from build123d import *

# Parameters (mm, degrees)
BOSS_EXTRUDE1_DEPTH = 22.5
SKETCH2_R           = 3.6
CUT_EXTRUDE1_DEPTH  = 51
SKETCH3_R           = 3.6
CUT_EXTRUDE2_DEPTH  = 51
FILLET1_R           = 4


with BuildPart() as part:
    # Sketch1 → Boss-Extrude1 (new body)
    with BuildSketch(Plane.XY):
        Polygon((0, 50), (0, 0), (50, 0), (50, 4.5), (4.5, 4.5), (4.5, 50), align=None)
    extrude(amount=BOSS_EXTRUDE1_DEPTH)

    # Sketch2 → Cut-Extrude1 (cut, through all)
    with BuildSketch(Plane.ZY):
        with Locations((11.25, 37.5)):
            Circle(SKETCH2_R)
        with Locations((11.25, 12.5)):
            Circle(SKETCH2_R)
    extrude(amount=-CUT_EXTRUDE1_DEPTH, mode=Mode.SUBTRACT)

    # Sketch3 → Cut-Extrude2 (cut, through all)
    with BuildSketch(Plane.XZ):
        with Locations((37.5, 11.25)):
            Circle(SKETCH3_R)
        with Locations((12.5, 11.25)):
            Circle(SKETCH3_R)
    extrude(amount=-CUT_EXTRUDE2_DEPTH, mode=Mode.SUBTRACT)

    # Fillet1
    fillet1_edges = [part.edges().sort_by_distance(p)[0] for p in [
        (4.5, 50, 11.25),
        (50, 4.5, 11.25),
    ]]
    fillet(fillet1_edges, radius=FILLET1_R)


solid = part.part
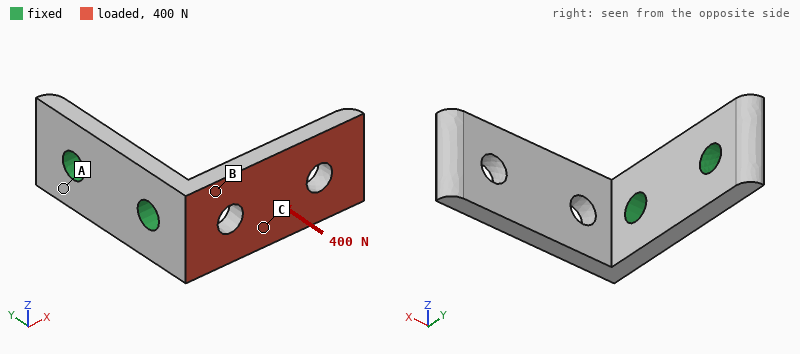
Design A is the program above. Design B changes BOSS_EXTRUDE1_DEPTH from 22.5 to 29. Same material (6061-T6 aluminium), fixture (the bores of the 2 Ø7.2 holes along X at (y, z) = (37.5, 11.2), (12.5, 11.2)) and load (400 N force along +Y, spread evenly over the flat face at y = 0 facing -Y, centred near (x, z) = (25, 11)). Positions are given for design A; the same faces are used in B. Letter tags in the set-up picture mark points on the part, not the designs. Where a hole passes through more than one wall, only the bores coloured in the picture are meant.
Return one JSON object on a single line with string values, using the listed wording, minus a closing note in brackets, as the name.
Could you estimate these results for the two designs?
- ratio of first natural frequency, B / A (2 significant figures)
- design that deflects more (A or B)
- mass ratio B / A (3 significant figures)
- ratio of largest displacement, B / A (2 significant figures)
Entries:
{"ratio of first natural frequency, B / A": "0.99", "design that deflects more": "A", "mass ratio B / A": "1.31", "ratio of largest displacement, B / A": "0.78"}
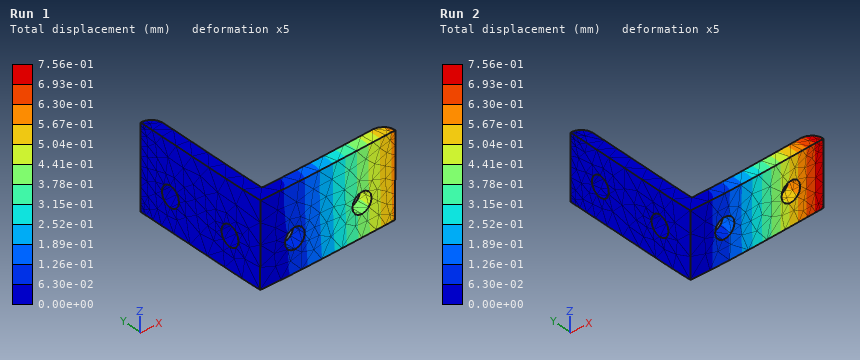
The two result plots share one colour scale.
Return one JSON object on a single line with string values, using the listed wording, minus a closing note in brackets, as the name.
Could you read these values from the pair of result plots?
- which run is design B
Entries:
{"which run is design B": "Run 1"}
